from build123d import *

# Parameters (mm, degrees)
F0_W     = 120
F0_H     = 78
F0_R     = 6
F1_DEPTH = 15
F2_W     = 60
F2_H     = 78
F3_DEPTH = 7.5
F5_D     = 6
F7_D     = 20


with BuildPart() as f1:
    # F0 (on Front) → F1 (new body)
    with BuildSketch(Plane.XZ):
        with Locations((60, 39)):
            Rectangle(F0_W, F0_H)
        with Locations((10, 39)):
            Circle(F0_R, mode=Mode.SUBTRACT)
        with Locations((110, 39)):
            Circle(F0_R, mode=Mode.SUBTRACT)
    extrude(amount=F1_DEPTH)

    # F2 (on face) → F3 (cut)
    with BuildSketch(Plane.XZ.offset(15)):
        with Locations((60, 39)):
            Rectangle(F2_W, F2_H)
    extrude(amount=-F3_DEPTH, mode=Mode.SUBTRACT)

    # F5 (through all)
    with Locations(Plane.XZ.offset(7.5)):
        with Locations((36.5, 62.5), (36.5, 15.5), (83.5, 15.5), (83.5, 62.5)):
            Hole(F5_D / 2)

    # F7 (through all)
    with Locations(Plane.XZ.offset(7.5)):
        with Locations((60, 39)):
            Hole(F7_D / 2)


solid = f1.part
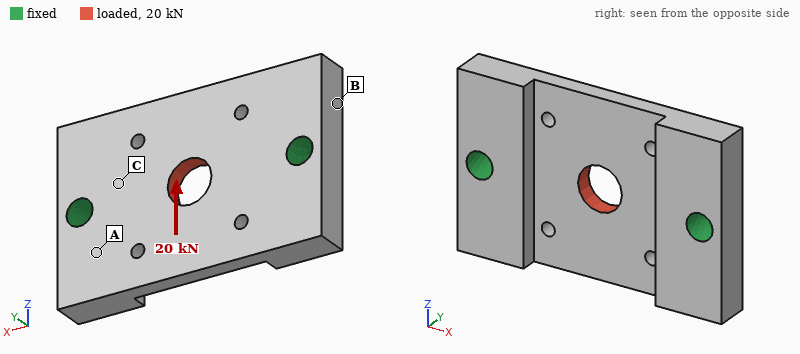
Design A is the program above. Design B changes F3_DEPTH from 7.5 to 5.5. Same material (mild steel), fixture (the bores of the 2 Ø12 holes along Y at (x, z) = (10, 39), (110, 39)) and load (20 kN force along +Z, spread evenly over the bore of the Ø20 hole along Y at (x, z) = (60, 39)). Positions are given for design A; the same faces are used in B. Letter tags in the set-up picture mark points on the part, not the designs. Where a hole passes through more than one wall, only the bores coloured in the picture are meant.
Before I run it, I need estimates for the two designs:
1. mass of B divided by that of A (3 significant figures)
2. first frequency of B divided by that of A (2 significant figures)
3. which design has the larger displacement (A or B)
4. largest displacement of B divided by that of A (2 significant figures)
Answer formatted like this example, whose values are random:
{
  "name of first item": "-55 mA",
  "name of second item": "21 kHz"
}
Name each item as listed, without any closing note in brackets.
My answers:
{
  "mass of B divided by that of A": "1.09",
  "first frequency of B divided by that of A": "0.98",
  "which design has the larger displacement": "A",
  "largest displacement of B divided by that of A": "0.82"
}
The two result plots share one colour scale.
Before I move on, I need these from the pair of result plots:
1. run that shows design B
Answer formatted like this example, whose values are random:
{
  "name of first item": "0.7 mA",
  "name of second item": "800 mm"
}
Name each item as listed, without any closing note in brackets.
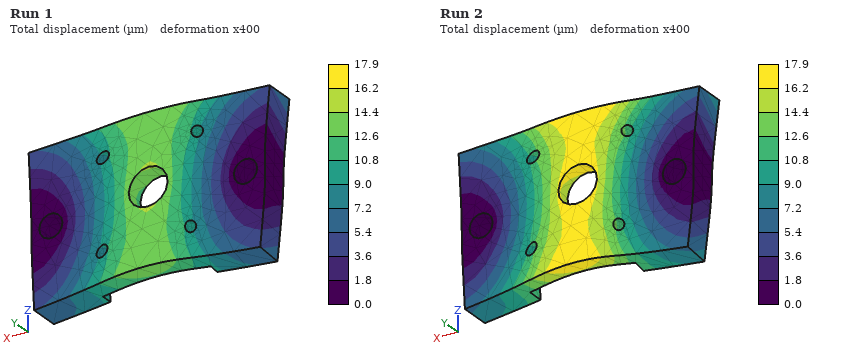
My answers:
{
  "run that shows design B": "Run 1"
}
